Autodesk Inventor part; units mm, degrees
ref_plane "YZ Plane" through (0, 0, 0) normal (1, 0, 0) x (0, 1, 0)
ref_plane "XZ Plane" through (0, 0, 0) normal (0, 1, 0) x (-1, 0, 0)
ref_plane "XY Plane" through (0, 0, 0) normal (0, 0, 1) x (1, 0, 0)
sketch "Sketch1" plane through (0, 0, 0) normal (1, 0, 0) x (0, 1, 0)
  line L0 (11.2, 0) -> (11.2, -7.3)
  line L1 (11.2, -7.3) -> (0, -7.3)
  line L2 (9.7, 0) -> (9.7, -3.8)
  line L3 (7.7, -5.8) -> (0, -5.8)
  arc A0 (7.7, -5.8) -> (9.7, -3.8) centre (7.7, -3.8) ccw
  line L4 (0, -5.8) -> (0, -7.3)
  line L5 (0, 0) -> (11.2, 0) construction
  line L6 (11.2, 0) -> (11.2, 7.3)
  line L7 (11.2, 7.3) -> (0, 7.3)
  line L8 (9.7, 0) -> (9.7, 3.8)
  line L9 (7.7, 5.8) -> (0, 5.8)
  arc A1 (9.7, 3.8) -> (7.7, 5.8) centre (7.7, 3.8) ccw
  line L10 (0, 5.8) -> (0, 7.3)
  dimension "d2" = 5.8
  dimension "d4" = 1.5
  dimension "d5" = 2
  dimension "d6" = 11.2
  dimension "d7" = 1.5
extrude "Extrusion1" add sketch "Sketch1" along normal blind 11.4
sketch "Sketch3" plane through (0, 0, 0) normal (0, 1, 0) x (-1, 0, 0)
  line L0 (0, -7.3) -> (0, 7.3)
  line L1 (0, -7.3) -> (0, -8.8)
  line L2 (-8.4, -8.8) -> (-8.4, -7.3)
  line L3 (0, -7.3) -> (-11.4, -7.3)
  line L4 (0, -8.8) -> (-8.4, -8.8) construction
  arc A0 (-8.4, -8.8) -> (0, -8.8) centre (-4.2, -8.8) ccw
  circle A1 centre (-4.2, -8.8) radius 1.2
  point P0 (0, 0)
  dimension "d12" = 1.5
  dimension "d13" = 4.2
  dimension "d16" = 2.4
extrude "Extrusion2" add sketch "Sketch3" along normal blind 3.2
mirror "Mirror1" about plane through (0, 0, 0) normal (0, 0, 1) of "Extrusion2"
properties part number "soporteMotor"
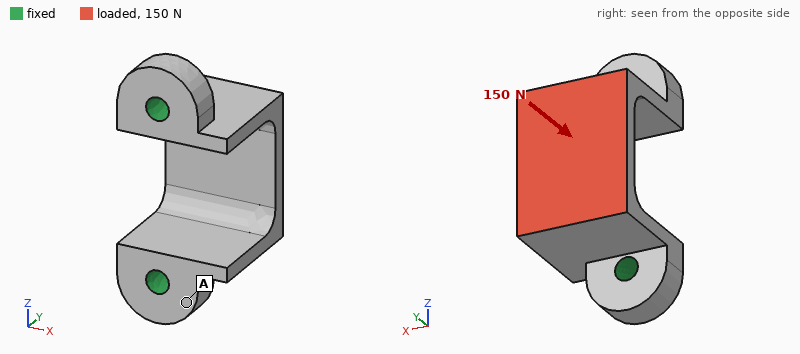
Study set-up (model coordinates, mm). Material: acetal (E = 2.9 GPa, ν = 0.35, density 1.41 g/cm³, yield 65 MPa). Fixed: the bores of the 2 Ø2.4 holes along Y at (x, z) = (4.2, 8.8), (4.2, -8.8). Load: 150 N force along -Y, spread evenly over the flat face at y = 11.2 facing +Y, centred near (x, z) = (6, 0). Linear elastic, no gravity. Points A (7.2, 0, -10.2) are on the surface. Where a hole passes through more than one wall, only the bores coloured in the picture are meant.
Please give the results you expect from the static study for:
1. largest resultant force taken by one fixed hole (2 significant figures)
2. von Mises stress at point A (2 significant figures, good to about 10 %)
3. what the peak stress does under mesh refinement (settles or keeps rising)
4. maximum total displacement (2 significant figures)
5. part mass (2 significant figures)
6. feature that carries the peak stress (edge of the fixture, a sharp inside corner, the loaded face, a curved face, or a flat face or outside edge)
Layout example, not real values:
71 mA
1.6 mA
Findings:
79 N
3.3 MPa
keeps rising
0.16 mm
1.2 g
edge of the fixture
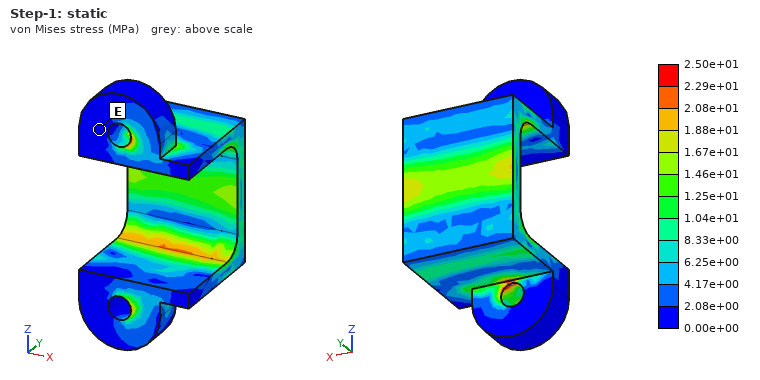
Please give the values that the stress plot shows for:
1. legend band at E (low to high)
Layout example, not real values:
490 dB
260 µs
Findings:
0.00e+00 to 2.08e+00 MPa
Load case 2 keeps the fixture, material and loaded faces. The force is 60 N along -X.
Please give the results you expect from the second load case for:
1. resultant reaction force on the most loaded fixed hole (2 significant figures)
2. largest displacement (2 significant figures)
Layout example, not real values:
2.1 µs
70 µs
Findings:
30 N
0.14 mm
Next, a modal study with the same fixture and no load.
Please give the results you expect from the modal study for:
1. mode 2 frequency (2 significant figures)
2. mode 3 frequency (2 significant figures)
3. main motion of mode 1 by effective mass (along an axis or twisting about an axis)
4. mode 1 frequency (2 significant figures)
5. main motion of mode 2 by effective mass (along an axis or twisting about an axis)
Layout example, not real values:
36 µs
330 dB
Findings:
5400 Hz
6900 Hz
along Z
4300 Hz
along X
